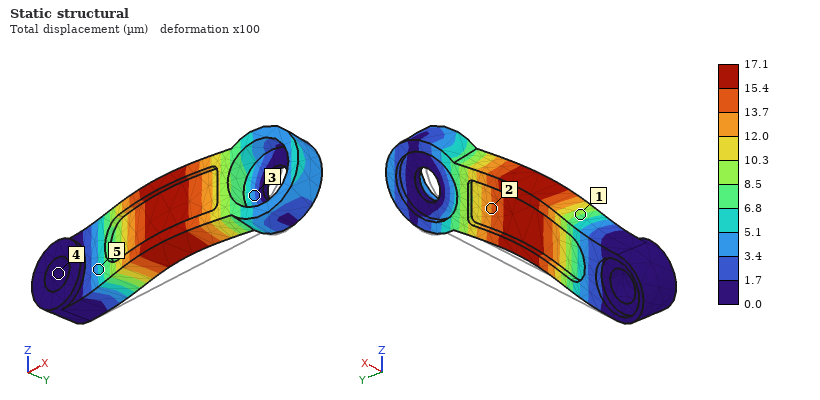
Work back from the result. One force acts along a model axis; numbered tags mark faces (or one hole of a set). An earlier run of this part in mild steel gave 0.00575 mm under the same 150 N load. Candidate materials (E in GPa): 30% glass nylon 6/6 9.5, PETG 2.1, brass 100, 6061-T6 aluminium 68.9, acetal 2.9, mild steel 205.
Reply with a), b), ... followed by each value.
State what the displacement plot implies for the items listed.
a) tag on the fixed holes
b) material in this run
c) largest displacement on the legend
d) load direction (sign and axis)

a) 4
b) 6061-T6 aluminium
c) 17.1 µm
d) -Y
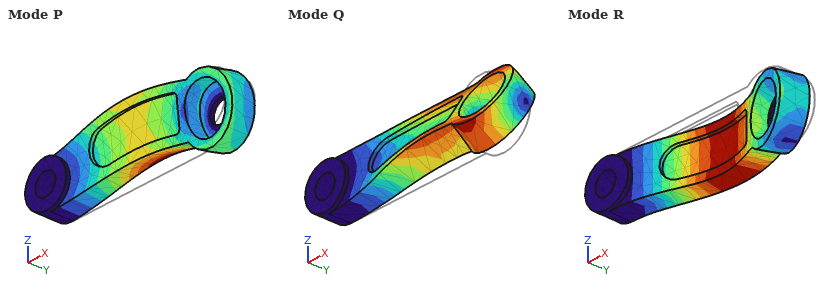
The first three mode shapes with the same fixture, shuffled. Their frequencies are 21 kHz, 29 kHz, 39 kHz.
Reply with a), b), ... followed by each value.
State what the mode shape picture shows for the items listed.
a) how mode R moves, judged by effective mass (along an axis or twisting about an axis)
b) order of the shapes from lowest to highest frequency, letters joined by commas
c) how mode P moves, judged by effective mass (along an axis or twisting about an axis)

a) along Y
b) R, Q, P
c) along Z
